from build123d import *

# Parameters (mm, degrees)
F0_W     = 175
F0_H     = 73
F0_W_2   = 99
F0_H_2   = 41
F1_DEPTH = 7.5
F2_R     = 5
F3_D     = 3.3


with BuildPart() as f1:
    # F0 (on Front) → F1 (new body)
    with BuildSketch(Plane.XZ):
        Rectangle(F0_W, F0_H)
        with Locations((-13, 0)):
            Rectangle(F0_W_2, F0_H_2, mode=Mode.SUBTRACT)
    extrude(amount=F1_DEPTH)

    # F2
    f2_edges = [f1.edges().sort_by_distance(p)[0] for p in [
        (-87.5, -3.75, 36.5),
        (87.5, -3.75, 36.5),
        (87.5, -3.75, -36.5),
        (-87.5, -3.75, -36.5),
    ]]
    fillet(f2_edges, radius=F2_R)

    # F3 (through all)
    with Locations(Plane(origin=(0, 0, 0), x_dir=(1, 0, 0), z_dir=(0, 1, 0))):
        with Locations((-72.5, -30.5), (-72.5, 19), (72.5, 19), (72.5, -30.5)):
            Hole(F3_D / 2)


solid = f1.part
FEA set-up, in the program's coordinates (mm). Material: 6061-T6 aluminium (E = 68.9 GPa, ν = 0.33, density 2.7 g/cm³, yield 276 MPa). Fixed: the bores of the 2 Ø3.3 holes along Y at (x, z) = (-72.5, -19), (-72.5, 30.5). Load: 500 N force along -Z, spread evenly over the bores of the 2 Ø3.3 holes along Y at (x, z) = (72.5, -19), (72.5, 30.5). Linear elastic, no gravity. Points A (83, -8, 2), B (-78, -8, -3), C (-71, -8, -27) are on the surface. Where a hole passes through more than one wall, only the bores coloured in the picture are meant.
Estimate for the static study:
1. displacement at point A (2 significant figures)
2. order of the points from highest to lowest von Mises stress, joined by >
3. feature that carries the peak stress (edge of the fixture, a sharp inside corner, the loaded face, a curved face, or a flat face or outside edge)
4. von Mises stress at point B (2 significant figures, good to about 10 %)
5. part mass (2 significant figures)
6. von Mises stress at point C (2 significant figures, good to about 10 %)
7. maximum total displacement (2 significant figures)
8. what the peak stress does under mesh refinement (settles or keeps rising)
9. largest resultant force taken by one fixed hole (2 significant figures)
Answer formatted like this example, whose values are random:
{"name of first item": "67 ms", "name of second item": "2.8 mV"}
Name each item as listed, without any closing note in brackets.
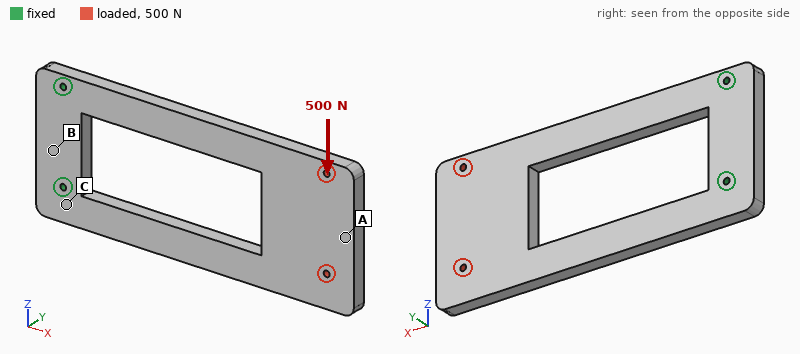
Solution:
{"displacement at point A": "0.26 mm", "order of the points from highest to lowest von Mises stress, joined by >": "C > B > A", "feature that carries the peak stress": "edge of the fixture", "von Mises stress at point B": "8.9 MPa", "part mass": "180 g", "von Mises stress at point C": "18 MPa", "maximum total displacement": "0.26 mm", "what the peak stress does under mesh refinement": "keeps rising", "largest resultant force taken by one fixed hole": "1.5 kN"}
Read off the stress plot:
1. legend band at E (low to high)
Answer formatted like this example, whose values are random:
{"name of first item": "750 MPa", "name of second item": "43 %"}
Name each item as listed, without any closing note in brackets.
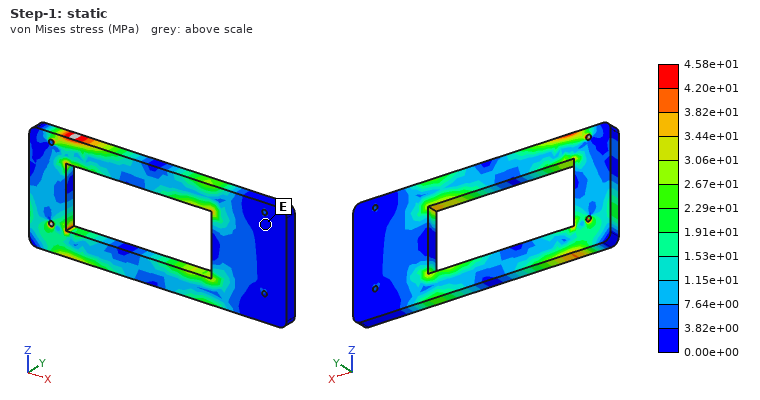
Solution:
{"legend band at E": "0.00e+00 to 3.82e+00 MPa"}
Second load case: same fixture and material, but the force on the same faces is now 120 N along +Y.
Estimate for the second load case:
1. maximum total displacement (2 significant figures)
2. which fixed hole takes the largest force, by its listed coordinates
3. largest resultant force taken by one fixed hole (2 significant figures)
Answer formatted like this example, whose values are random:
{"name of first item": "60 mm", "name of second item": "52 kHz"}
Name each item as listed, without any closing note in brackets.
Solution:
{"maximum total displacement": "1.8 mm", "which fixed hole takes the largest force, by its listed coordinates": "(-72.5, 30.5)", "largest resultant force taken by one fixed hole": "86 N"}
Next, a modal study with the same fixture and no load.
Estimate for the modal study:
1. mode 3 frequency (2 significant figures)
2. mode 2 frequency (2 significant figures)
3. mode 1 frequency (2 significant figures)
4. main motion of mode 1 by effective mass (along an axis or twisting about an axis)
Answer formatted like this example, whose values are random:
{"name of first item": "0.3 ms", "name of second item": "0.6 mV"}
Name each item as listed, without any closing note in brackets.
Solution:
{"mode 3 frequency": "740 Hz", "mode 2 frequency": "720 Hz", "mode 1 frequency": "170 Hz", "main motion of mode 1 by effective mass": "along Y"}
